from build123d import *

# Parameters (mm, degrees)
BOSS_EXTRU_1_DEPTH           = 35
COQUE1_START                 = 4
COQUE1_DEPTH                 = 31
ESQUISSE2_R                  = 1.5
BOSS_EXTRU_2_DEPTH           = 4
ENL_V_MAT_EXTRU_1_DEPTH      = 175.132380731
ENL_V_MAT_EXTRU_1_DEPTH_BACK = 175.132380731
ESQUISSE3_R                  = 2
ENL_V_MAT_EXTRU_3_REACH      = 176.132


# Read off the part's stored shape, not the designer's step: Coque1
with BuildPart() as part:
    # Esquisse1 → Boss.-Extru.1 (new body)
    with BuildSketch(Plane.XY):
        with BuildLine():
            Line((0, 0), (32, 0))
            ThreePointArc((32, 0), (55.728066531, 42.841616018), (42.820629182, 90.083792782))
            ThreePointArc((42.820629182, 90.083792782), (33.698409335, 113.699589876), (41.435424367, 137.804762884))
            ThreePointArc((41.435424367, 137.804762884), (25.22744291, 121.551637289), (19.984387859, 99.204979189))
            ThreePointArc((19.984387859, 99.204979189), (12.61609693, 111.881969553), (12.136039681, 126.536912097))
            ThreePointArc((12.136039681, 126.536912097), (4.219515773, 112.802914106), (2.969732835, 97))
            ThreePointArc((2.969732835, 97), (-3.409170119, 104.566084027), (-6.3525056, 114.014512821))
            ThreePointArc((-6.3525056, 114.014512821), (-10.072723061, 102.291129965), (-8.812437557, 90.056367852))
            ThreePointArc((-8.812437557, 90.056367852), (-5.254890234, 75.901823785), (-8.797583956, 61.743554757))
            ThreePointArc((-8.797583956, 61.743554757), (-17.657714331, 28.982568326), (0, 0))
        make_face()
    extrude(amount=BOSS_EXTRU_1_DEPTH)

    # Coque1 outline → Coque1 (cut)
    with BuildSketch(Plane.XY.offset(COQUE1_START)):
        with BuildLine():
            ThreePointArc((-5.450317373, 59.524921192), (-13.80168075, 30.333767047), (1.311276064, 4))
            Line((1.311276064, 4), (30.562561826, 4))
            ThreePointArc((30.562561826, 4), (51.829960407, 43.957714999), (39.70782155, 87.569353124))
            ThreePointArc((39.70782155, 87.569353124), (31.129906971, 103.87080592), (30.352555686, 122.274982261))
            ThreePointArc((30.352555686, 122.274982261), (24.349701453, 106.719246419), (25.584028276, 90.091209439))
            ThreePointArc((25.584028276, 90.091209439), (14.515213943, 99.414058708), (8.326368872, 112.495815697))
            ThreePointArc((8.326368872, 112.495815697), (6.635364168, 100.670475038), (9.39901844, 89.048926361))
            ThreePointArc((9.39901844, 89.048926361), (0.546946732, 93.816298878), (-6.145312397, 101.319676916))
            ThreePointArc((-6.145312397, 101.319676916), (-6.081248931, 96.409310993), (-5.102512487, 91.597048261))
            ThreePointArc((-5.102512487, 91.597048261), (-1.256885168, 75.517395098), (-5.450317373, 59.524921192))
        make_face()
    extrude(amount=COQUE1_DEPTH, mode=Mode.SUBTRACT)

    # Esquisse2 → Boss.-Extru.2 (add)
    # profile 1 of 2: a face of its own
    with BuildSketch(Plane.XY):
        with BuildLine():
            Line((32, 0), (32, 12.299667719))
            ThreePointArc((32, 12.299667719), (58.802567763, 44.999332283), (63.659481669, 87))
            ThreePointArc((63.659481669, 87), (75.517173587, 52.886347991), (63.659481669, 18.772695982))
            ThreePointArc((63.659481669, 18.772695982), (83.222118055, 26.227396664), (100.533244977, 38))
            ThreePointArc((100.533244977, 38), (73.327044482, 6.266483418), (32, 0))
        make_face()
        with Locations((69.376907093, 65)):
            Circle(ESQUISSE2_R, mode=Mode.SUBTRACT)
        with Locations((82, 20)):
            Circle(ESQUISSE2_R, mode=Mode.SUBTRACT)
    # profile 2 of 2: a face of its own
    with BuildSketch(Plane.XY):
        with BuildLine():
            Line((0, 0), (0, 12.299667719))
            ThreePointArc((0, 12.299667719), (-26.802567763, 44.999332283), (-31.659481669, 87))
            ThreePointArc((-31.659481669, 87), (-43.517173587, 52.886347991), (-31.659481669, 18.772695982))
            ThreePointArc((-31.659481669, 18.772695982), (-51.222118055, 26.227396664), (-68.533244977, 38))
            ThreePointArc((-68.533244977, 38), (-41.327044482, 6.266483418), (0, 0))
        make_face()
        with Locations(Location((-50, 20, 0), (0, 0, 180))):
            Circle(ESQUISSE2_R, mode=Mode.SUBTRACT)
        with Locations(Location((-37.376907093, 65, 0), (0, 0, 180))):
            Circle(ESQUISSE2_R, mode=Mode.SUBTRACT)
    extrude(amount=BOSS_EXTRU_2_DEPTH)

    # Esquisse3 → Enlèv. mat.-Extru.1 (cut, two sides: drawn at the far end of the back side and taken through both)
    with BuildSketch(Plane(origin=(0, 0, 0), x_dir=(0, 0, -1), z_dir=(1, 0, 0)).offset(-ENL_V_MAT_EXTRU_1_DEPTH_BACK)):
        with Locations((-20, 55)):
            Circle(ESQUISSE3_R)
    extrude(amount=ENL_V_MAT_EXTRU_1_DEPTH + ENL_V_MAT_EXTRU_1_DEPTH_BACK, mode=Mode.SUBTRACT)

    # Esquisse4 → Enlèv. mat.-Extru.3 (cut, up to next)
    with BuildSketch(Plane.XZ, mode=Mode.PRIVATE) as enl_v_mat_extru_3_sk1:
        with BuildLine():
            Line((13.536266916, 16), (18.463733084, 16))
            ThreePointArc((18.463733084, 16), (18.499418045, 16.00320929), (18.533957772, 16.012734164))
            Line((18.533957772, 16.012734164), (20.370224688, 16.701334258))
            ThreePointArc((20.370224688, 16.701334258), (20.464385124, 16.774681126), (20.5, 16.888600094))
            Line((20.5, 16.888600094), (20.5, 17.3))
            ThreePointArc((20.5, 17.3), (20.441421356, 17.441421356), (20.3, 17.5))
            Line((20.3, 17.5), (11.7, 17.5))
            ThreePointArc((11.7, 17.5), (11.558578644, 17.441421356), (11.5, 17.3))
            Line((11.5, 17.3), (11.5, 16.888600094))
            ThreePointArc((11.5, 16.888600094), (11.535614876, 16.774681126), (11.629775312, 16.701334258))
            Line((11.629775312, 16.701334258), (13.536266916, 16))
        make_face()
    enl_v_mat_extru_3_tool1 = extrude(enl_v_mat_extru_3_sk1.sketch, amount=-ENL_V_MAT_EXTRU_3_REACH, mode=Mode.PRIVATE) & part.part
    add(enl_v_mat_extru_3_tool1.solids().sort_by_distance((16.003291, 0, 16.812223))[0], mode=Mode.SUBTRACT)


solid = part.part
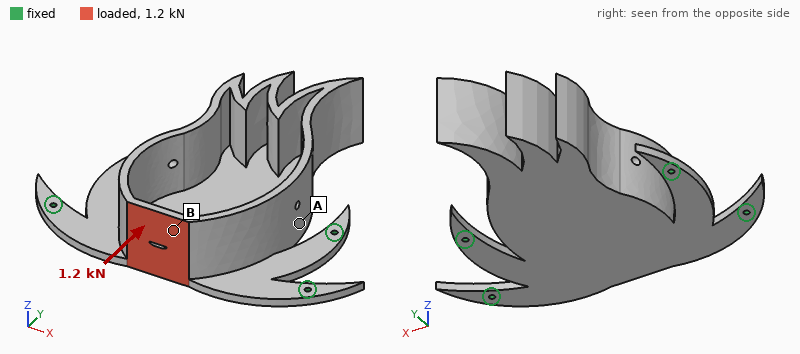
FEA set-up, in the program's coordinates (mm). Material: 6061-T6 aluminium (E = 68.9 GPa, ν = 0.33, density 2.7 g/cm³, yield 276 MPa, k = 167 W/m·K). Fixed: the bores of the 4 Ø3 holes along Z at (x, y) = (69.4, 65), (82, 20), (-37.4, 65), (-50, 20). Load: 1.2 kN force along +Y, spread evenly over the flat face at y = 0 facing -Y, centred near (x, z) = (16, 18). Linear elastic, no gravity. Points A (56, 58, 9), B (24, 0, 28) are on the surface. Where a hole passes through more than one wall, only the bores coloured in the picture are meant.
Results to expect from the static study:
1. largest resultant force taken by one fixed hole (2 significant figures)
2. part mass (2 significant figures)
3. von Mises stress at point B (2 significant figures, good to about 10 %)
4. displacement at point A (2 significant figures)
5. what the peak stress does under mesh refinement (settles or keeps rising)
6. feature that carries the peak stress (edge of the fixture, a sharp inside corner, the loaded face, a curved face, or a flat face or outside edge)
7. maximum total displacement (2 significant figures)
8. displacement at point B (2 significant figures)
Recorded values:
600 N
240 g
29 MPa
0.32 mm
keeps rising
edge of the fixture
1.3 mm
0.52 mm
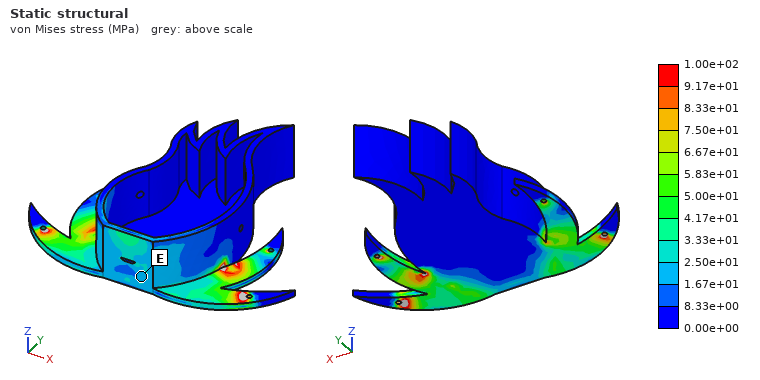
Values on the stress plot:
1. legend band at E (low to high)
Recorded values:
1.67e+01 to 2.50e+01 MPa
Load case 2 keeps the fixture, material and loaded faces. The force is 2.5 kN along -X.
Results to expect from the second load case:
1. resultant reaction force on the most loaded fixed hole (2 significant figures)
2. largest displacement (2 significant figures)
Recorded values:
1.2 kN
0.20 mm
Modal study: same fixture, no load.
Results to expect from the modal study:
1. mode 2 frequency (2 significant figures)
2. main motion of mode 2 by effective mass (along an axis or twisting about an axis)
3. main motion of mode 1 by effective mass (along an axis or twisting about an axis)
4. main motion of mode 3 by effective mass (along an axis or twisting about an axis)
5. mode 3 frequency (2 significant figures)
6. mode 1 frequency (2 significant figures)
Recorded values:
870 Hz
along Z
along Z
along X
1100 Hz
230 Hz
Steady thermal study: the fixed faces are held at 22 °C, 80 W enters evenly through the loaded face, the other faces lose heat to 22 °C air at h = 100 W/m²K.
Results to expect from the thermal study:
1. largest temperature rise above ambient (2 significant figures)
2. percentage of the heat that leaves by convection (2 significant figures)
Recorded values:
56 K
78 %
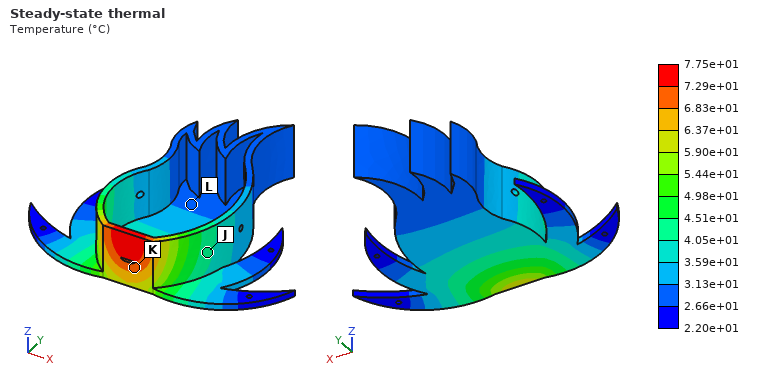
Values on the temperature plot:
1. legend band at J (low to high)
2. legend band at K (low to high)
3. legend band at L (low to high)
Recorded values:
4.05e+01 to 4.51e+01 °C
6.83e+01 to 7.29e+01 °C
2.66e+01 to 3.13e+01 °C
